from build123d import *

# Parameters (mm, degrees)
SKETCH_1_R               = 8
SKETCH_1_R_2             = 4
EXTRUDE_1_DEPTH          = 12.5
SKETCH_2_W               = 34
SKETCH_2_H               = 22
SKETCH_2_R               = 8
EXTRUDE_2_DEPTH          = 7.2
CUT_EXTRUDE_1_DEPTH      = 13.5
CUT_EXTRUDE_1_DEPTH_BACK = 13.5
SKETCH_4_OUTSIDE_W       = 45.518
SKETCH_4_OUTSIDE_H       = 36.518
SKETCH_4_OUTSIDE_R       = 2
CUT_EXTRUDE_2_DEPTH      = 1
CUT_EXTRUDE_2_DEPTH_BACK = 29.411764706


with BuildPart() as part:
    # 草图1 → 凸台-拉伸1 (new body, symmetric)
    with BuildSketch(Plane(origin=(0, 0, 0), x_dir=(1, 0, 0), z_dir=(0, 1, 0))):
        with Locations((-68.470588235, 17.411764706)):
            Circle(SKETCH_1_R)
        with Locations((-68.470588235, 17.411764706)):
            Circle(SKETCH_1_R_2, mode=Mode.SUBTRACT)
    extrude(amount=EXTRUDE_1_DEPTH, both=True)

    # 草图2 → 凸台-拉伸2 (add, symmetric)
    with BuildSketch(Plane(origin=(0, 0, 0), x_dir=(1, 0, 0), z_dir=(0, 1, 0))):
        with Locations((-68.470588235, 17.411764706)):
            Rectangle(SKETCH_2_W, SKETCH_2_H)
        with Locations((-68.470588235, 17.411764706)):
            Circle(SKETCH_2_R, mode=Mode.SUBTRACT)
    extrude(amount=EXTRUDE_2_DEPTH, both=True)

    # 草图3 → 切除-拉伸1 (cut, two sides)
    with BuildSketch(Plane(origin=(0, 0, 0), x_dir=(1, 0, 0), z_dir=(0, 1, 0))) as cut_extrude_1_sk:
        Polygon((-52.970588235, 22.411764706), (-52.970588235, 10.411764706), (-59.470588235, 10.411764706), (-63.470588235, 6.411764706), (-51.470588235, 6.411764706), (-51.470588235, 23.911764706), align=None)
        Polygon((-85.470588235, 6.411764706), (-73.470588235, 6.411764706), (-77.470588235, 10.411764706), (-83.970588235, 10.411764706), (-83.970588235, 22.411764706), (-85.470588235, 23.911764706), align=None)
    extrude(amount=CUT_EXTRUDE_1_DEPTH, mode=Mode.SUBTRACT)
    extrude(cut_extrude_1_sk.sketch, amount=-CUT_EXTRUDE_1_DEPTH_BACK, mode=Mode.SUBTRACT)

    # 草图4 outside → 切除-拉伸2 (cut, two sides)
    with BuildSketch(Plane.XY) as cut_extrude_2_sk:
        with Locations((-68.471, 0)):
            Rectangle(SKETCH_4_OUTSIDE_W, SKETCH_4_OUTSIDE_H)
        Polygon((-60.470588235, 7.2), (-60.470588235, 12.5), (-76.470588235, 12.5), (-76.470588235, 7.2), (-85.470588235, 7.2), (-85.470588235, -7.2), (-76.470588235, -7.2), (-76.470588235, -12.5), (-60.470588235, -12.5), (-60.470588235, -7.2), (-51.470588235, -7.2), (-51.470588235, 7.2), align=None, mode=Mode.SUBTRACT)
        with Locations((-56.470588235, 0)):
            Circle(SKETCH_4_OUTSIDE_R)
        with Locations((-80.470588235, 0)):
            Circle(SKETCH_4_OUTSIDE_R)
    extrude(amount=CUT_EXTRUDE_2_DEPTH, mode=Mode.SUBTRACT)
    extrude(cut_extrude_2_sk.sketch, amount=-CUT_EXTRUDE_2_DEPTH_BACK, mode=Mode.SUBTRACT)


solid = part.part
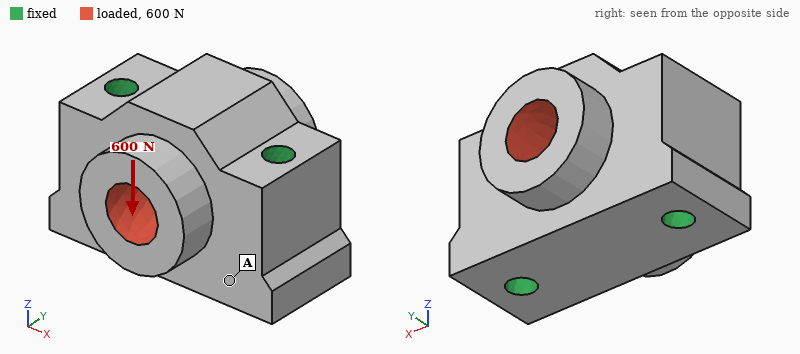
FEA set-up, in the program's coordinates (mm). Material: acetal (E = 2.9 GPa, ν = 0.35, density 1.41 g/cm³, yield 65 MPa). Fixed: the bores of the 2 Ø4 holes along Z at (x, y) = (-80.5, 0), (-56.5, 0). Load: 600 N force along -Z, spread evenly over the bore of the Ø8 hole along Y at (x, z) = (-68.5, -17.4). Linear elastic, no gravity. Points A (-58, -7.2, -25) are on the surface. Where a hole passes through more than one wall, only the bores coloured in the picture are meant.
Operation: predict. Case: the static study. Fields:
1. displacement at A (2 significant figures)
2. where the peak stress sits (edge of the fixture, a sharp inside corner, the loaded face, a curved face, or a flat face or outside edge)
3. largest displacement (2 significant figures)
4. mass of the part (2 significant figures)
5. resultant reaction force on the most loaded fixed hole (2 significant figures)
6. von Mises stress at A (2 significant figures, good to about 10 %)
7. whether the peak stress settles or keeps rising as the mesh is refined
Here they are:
3.7 µm
edge of the fixture
18 µm
13 g
300 N
0.92 MPa
keeps rising
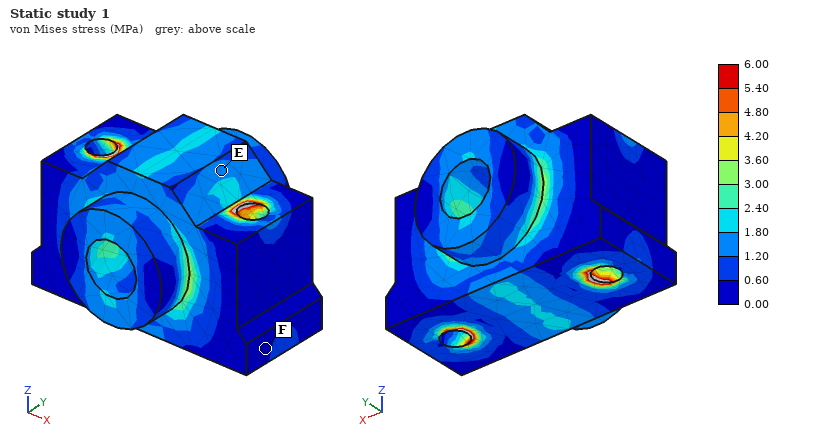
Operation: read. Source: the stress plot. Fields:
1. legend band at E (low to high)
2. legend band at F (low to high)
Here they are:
1.20 to 1.80 MPa
0.00 to 0.60 MPa
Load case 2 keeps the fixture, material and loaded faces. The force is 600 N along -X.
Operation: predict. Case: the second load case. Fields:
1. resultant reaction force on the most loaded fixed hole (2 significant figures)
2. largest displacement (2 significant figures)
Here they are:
300 N
12 µm
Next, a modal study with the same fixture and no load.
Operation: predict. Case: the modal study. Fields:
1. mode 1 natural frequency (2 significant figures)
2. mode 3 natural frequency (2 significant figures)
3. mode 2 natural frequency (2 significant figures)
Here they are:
10 kHz
13 kHz
13 kHz
